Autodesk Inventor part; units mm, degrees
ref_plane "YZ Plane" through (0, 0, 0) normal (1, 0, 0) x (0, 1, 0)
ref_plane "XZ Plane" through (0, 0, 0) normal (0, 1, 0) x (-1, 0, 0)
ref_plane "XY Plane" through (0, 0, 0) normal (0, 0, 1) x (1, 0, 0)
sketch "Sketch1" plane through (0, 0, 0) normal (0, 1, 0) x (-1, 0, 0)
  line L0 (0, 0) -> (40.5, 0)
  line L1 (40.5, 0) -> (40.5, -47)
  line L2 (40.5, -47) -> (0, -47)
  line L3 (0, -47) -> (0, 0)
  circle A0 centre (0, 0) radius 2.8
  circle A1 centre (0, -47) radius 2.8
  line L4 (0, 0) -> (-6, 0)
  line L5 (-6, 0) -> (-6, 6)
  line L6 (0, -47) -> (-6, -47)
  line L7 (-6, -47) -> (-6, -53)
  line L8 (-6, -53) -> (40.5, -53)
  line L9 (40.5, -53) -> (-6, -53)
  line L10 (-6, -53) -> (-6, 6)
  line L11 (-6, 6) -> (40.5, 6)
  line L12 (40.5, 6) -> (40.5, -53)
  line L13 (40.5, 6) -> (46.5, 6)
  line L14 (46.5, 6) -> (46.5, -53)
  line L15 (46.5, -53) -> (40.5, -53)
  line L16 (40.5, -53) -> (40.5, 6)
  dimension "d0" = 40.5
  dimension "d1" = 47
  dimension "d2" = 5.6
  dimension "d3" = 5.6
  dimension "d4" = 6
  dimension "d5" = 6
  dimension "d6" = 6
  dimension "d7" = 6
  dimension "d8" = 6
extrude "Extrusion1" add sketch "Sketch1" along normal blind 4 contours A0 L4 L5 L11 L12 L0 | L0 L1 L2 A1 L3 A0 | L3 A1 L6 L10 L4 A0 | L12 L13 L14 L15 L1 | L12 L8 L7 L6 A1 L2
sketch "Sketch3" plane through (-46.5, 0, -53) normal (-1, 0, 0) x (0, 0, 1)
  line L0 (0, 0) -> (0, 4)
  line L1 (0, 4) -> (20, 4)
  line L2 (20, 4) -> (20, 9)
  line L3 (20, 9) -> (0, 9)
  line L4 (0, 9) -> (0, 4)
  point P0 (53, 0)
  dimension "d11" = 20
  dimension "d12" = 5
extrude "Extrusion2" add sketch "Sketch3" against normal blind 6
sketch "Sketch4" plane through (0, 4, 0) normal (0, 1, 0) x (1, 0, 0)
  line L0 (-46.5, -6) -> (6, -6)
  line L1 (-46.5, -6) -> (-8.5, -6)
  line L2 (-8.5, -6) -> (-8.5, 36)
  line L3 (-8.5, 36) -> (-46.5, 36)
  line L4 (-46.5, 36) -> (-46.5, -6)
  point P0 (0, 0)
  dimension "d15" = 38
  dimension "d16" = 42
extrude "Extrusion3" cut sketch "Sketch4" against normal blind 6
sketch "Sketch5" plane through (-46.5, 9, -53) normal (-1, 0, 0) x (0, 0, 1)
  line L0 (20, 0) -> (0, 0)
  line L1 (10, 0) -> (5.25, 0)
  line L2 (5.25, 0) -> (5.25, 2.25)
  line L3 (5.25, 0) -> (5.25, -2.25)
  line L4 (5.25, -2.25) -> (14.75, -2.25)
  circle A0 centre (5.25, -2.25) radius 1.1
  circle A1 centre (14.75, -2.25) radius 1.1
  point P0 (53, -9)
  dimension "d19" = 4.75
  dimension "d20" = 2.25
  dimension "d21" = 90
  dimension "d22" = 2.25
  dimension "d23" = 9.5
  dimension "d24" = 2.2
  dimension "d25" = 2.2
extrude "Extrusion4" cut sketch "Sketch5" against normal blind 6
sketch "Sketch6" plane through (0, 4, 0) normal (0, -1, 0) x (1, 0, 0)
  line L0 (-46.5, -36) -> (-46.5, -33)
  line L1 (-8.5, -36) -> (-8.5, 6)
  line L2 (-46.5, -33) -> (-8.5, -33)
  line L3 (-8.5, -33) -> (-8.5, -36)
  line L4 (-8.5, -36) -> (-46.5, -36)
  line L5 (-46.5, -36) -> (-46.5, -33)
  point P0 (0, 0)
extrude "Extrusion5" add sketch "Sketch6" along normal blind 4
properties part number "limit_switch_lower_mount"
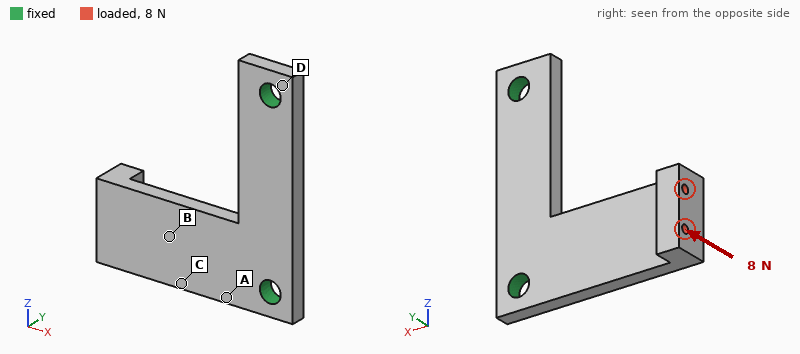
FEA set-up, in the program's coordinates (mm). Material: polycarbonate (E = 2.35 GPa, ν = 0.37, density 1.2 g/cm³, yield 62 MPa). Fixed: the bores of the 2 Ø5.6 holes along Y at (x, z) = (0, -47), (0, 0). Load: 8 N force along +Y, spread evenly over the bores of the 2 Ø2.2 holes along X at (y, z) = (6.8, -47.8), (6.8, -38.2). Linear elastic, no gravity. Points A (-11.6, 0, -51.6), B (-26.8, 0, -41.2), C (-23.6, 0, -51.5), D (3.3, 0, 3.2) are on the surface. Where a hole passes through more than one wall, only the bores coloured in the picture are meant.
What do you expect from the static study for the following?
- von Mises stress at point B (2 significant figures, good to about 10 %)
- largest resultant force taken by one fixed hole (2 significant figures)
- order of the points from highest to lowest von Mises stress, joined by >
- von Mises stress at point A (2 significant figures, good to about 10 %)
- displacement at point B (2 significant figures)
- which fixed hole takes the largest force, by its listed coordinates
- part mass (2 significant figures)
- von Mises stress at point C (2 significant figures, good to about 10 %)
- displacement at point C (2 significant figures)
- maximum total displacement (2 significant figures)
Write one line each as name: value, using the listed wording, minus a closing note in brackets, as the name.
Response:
von Mises stress at point B: 2.4 MPa
largest resultant force taken by one fixed hole: 8.7 N
order of the points from highest to lowest von Mises stress, joined by >: A > C > B > D
von Mises stress at point A: 5.0 MPa
displacement at point B: 0.36 mm
which fixed hole takes the largest force, by its listed coordinates: (0, -47)
part mass: 8.2 g
von Mises stress at point C: 3.0 MPa
displacement at point C: 0.26 mm
maximum total displacement: 0.91 mm
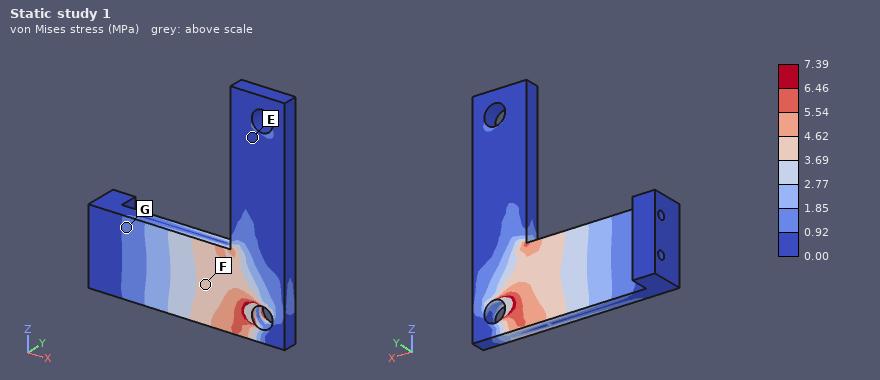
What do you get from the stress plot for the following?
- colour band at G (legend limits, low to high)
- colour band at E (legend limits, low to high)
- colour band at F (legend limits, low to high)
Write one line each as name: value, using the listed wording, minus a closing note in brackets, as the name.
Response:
colour band at G: 0.92 to 1.85 MPa
colour band at E: 0.00 to 0.92 MPa
colour band at F: 3.69 to 4.62 MPa
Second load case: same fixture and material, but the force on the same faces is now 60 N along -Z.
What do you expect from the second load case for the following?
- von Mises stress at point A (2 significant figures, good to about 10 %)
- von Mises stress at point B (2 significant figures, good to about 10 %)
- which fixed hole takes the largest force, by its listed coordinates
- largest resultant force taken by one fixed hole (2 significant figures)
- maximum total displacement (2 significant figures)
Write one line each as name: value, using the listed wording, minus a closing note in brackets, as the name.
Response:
von Mises stress at point A: 7.5 MPa
von Mises stress at point B: 3.2 MPa
which fixed hole takes the largest force, by its listed coordinates: (0, 0)
largest resultant force taken by one fixed hole: 56 N
maximum total displacement: 0.74 mm
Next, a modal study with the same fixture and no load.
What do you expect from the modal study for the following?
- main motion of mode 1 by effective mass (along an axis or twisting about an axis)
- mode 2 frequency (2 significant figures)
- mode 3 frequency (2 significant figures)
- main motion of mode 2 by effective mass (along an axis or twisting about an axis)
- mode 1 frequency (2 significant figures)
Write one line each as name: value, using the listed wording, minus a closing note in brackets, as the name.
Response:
main motion of mode 1 by effective mass: along Y
mode 2 frequency: 1300 Hz
mode 3 frequency: 1600 Hz
main motion of mode 2 by effective mass: along Z
mode 1 frequency: 360 Hz
